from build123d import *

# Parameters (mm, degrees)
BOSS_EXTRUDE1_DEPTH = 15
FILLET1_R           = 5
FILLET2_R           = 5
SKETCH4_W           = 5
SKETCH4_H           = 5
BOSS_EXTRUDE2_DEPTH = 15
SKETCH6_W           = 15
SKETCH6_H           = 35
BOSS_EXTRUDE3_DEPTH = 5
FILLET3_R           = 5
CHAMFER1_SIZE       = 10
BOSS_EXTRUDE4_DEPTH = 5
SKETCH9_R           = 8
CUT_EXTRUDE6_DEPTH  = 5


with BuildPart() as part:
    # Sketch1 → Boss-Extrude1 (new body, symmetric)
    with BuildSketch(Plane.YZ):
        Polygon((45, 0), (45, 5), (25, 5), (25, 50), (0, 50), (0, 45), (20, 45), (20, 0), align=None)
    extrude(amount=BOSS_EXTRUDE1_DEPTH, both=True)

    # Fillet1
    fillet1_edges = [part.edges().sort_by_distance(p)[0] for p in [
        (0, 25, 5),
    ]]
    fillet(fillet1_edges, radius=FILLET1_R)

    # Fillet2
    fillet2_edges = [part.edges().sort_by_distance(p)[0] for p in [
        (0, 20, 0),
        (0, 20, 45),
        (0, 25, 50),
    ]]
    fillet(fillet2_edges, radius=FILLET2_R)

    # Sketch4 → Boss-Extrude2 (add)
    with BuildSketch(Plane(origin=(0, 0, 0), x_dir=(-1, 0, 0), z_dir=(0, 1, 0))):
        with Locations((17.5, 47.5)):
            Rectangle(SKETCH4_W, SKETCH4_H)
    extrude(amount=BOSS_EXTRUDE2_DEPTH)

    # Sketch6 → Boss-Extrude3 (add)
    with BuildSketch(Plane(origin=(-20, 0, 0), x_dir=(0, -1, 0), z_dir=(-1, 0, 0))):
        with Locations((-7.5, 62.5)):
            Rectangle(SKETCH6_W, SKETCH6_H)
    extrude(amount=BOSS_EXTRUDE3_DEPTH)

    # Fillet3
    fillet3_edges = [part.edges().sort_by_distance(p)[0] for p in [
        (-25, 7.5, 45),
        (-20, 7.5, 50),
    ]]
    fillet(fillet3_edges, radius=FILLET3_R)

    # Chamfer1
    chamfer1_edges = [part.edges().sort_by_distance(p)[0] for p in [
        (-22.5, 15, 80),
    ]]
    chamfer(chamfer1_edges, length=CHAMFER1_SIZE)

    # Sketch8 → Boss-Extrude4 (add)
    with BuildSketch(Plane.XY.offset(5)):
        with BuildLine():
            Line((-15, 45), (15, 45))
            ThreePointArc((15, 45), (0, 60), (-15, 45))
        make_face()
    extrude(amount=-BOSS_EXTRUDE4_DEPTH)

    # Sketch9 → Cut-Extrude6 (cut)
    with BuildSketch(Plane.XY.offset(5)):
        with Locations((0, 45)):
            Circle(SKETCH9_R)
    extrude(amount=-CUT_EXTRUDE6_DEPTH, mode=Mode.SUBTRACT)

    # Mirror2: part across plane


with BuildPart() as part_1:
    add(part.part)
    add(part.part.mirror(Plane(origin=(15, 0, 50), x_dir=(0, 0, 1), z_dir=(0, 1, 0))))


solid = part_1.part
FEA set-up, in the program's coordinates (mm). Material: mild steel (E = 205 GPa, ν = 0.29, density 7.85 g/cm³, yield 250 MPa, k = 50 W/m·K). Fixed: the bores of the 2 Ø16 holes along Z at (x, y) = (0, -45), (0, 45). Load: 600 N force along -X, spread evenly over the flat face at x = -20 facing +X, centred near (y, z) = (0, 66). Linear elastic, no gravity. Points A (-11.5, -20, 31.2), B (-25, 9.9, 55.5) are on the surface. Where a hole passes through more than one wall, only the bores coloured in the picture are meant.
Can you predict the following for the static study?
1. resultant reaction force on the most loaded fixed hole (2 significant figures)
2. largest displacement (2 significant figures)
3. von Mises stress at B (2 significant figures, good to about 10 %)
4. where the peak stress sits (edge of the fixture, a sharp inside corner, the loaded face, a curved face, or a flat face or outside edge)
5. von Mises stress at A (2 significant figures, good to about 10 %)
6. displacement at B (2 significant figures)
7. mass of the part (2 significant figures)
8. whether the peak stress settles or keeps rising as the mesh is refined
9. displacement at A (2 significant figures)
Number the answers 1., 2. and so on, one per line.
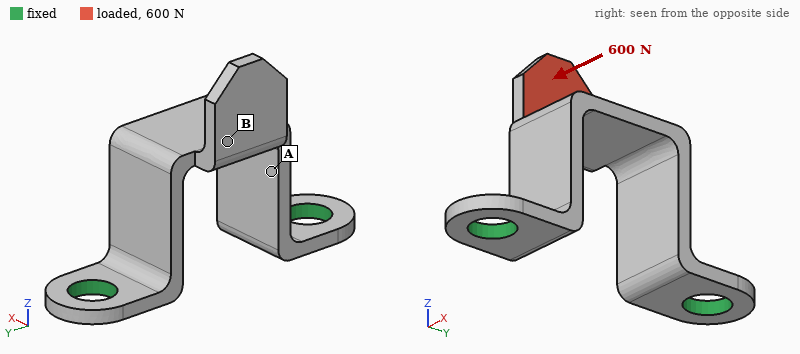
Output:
1. 300 N
2. 0.25 mm
3. 47 MPa
4. a sharp inside corner
5. 19 MPa
6. 0.14 mm
7. 270 g
8. keeps rising
9. 0.055 mm
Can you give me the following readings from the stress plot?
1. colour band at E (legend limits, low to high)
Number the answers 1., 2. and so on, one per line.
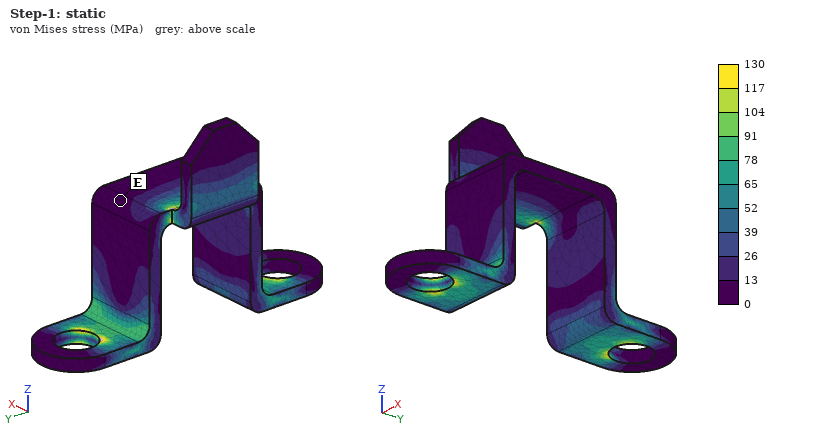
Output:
1. 0 to 13 MPa
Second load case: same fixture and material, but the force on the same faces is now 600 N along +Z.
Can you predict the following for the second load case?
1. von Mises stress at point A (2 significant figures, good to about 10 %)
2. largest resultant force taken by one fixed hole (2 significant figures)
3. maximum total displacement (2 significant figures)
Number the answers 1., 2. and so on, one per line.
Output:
1. 17 MPa
2. 320 N
3. 76 µm
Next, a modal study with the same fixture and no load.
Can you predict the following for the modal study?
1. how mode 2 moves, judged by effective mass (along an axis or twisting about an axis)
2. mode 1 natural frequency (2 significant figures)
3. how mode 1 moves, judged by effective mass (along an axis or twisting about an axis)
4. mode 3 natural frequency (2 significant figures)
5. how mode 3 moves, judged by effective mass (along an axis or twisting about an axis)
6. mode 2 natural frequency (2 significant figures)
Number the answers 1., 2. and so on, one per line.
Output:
1. along Y
2. 1200 Hz
3. along X
4. 2600 Hz
5. twisting about Z
6. 1600 Hz
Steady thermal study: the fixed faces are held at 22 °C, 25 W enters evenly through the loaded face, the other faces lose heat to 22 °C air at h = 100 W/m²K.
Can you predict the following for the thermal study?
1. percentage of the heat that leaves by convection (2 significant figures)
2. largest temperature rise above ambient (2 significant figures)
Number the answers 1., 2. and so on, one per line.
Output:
1. 89 %
2. 83 K
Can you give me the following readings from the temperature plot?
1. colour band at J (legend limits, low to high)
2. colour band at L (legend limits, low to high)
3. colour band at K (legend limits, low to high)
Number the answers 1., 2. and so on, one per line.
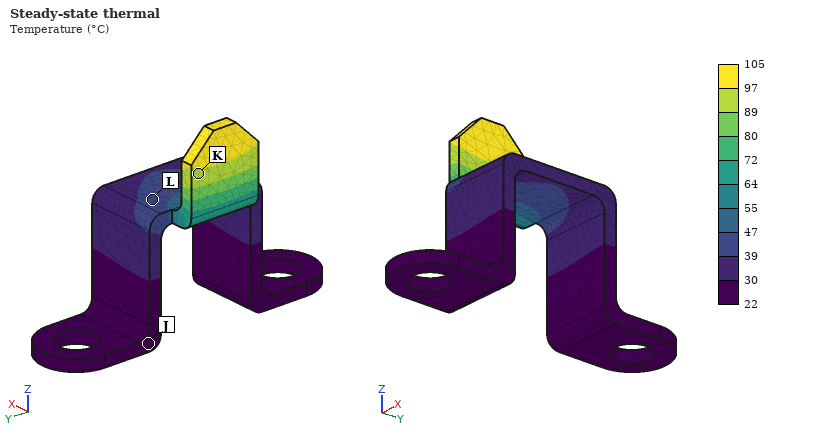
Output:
1. 22 to 30 °C
2. 39 to 47 °C
3. 89 to 97 °C
